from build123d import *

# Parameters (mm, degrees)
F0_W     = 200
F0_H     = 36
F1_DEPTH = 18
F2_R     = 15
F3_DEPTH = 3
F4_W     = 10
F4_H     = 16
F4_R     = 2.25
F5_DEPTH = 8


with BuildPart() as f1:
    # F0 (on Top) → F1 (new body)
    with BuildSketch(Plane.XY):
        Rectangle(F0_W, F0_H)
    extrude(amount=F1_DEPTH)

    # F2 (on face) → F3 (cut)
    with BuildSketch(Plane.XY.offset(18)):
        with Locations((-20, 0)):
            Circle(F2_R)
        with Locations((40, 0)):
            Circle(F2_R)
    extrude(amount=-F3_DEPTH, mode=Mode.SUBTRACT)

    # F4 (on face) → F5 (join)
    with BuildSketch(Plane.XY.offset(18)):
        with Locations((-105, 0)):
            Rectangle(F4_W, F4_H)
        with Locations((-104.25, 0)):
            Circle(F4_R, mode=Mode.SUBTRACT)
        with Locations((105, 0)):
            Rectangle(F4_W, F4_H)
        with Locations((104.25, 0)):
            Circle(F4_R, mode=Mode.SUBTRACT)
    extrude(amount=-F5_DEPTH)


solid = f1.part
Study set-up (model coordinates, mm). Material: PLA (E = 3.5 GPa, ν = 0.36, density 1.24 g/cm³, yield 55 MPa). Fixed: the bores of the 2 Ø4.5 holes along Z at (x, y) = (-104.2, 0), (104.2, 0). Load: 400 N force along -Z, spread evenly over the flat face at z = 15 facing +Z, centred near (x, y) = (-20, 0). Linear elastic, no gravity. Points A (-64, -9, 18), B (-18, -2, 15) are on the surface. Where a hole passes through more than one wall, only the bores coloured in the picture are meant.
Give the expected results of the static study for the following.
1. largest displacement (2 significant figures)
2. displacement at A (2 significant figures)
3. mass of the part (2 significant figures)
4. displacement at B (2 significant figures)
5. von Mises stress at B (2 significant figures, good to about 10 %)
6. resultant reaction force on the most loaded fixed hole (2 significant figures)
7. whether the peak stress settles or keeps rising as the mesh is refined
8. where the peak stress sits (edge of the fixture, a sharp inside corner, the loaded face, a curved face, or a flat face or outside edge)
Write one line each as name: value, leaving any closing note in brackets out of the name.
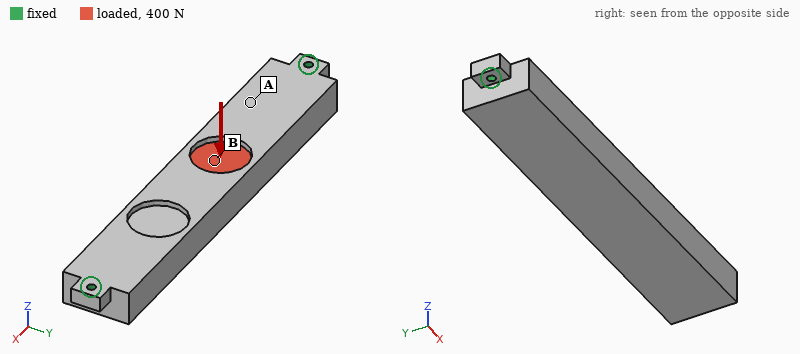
largest displacement: 0.73 mm
displacement at A: 0.38 mm
mass of the part: 160 g
displacement at B: 0.71 mm
von Mises stress at B: 5.6 MPa
resultant reaction force on the most loaded fixed hole: 680 N
whether the peak stress settles or keeps rising as the mesh is refined: keeps rising
where the peak stress sits: edge of the fixture
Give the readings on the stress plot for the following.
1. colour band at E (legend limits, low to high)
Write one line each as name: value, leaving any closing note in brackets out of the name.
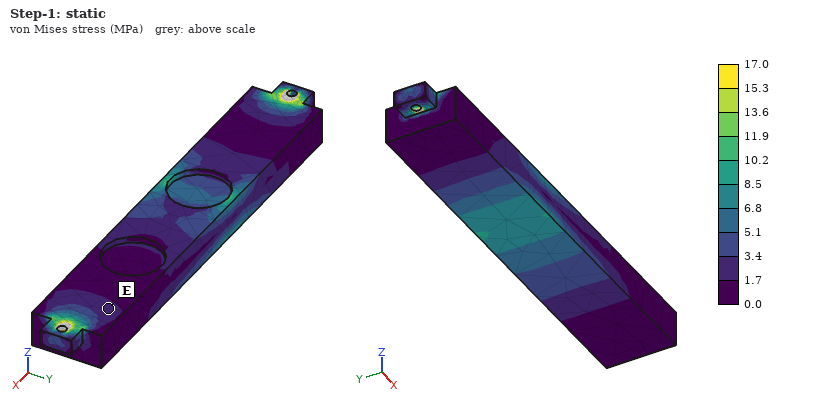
colour band at E: 1.7 to 3.4 MPa
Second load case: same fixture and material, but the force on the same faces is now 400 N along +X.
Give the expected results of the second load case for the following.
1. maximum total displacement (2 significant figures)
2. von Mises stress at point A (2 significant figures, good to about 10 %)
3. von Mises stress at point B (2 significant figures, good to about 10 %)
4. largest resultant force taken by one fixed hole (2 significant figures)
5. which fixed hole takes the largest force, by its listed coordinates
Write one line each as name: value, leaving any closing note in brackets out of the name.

maximum total displacement: 39 µm
von Mises stress at point A: 0.96 MPa
von Mises stress at point B: 0.93 MPa
largest resultant force taken by one fixed hole: 240 N
which fixed hole takes the largest force, by its listed coordinates: (-104.2, 0)
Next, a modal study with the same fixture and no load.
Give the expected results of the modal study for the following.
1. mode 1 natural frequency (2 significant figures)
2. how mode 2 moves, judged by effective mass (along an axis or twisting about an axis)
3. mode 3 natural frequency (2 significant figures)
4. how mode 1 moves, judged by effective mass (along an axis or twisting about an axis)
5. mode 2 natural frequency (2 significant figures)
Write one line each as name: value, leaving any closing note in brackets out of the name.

mode 1 natural frequency: 430 Hz
how mode 2 moves, judged by effective mass: along Y
mode 3 natural frequency: 940 Hz
how mode 1 moves, judged by effective mass: along Z
mode 2 natural frequency: 620 Hz
